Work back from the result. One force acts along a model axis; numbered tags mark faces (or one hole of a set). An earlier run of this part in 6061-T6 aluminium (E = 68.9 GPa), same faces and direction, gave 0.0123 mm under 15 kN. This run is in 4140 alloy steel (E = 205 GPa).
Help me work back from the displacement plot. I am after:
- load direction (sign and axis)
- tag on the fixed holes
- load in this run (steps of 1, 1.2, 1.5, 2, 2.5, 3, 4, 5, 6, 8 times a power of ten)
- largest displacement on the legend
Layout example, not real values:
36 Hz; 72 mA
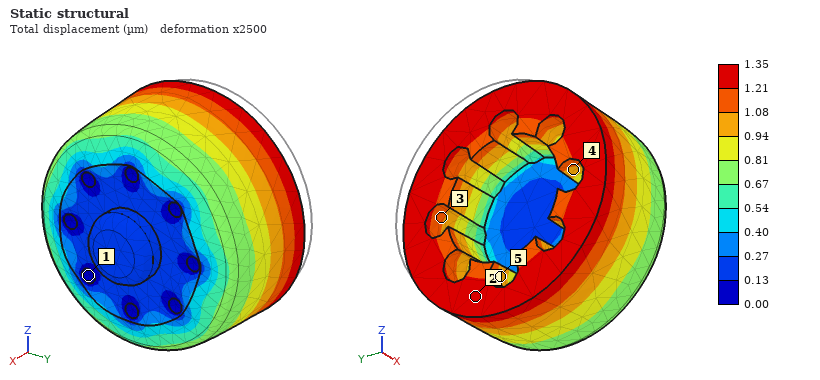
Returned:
+X; 1; 5 kN; 1.35 µm
